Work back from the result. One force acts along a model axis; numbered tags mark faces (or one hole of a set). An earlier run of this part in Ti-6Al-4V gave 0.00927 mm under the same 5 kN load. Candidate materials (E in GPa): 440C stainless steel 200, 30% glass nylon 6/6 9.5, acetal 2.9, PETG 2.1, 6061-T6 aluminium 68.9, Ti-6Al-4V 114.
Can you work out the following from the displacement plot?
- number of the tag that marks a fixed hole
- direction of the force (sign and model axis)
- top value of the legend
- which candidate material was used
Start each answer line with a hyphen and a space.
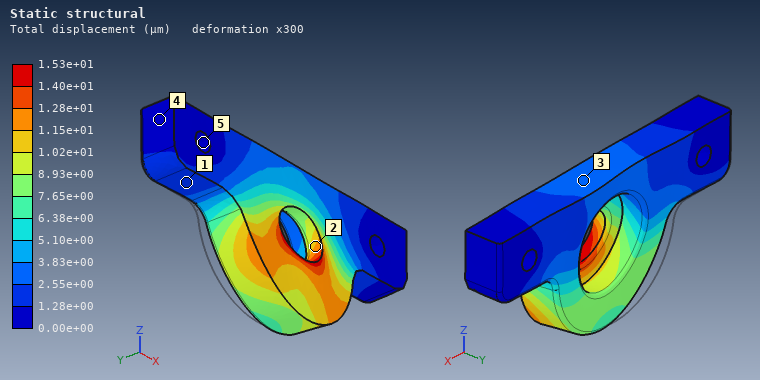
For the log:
- 5
- +X
- 1.53e+01 µm
- 6061-T6 aluminium
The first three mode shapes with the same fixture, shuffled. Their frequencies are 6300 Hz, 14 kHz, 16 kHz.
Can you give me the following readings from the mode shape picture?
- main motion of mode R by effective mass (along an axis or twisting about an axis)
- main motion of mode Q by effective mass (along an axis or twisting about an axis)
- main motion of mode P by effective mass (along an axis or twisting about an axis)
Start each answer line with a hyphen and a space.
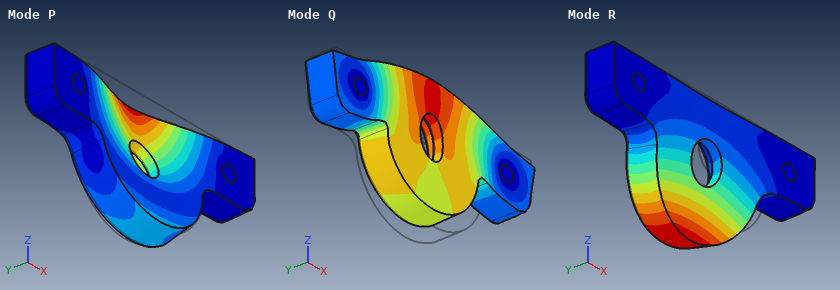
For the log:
- along Y
- along Z
- along Y
